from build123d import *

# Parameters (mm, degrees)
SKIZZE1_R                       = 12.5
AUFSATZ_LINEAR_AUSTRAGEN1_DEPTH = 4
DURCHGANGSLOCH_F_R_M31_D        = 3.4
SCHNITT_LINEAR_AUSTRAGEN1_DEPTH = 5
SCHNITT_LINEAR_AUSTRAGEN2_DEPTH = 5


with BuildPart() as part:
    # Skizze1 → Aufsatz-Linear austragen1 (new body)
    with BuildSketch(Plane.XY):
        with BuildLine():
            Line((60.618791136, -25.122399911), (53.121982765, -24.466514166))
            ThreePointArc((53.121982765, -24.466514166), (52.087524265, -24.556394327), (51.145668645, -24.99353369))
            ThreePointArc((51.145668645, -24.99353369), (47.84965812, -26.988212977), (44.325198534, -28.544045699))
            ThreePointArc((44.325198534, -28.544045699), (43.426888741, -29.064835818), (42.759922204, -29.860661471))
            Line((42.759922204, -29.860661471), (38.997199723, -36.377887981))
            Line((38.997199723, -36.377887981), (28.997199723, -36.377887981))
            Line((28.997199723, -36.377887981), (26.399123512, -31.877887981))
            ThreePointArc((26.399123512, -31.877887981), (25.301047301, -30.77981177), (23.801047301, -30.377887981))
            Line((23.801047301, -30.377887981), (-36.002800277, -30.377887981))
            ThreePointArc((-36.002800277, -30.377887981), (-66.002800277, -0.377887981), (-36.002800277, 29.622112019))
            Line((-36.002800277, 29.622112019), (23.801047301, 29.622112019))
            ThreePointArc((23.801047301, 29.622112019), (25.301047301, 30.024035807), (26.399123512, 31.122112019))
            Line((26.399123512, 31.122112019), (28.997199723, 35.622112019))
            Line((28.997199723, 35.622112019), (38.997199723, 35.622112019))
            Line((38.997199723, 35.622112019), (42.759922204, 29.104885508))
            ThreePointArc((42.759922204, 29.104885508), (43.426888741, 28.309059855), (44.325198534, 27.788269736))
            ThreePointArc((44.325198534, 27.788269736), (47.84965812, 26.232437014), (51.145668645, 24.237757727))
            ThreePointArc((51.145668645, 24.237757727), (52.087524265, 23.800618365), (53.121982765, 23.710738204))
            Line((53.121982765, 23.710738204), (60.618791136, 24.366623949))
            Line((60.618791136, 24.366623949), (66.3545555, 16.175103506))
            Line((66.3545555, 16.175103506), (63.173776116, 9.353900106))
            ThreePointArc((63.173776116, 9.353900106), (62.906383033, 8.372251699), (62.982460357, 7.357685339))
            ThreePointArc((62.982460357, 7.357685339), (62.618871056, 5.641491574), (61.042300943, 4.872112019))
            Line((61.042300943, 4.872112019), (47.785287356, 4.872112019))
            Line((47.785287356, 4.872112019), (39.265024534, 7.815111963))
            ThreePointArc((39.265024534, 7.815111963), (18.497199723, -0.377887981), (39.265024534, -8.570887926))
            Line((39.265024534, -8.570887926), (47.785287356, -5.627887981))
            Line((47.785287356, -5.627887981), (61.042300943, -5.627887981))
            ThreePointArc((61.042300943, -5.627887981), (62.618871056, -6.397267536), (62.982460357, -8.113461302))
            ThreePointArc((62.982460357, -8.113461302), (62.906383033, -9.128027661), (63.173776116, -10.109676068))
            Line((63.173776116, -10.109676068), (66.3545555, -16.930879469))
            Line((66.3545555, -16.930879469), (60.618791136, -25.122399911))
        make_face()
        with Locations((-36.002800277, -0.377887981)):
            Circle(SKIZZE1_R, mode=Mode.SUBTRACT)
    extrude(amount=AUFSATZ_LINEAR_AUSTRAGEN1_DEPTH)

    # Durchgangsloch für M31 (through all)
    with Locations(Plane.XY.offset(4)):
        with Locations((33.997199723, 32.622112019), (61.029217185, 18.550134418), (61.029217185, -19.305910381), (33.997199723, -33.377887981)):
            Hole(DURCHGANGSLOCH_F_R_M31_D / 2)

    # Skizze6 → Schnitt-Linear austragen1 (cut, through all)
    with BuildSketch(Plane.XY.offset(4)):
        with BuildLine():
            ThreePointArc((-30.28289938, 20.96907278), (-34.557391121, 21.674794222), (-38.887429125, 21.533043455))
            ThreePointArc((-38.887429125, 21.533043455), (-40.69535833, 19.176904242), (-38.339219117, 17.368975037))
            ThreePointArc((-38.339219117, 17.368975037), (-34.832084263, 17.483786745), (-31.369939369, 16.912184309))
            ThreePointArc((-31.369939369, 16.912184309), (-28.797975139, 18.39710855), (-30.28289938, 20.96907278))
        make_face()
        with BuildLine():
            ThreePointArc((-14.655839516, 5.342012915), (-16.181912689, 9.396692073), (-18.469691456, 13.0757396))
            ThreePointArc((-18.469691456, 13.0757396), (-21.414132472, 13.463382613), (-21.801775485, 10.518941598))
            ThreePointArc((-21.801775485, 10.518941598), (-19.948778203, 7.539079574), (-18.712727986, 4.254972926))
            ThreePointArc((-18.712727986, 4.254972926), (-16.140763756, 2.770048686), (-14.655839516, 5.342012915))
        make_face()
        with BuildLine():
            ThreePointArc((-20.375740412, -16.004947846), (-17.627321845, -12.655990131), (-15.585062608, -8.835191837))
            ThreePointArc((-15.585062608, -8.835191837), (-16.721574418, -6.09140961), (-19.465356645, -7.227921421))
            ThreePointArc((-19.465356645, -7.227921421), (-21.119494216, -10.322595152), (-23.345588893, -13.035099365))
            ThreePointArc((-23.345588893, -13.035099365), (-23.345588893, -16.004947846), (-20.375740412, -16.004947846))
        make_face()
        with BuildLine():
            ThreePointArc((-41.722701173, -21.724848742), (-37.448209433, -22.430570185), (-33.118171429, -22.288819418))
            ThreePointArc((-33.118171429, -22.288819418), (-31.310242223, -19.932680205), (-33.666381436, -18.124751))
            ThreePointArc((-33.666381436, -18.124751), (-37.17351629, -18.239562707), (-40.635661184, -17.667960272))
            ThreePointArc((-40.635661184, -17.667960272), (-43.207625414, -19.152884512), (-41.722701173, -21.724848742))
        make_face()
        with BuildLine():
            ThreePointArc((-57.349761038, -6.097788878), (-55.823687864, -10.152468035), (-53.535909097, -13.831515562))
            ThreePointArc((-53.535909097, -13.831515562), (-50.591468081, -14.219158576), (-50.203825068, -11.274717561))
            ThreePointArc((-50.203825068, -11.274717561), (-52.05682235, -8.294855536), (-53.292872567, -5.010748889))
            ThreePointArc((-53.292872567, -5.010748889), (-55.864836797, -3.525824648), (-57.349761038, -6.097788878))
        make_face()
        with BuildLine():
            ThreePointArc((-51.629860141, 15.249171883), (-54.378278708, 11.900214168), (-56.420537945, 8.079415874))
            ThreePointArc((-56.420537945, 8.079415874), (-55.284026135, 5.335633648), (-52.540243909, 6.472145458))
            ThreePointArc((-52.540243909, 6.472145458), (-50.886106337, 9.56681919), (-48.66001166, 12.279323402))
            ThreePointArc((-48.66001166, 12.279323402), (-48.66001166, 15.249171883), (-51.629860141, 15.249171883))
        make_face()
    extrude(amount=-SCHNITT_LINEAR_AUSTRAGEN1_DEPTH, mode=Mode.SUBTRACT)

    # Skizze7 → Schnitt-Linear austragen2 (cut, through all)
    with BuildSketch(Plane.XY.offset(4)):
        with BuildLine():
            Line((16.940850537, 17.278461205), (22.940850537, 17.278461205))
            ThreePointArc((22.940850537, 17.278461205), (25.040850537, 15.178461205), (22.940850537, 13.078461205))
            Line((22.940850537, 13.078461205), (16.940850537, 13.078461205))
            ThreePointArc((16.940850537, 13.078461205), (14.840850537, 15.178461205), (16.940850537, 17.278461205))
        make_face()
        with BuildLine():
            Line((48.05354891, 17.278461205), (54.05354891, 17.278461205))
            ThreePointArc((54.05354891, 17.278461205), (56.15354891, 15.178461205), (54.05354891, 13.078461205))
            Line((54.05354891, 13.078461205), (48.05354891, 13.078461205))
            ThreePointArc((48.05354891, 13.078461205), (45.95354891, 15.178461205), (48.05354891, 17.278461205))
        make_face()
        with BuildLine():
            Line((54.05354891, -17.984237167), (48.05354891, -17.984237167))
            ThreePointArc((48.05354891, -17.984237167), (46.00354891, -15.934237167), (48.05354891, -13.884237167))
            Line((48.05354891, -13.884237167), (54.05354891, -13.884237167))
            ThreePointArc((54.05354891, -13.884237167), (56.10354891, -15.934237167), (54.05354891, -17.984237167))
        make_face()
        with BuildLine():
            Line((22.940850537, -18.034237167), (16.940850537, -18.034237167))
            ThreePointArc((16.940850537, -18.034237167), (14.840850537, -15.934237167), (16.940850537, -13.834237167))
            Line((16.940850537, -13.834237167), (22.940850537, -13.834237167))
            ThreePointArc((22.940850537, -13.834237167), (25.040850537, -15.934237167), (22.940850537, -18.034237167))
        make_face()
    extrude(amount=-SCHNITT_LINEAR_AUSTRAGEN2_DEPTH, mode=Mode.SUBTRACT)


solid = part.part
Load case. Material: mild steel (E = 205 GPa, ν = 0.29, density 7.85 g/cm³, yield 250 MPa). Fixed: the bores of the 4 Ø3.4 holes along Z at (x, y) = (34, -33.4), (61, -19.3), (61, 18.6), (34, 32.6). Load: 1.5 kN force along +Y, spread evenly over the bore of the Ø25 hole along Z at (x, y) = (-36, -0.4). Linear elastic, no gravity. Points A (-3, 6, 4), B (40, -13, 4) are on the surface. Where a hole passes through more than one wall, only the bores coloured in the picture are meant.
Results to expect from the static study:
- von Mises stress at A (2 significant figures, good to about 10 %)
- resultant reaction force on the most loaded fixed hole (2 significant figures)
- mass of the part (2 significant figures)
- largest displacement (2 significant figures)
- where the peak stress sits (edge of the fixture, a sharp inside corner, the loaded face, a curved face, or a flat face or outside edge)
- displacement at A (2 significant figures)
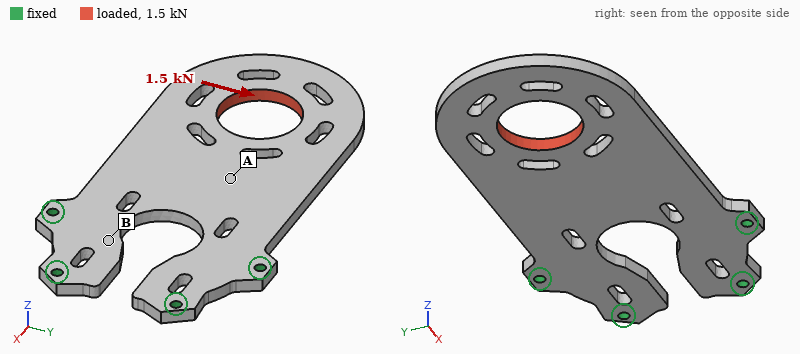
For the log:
20 MPa
1.6 kN
180 g
38 µm
a curved face
9.6 µm
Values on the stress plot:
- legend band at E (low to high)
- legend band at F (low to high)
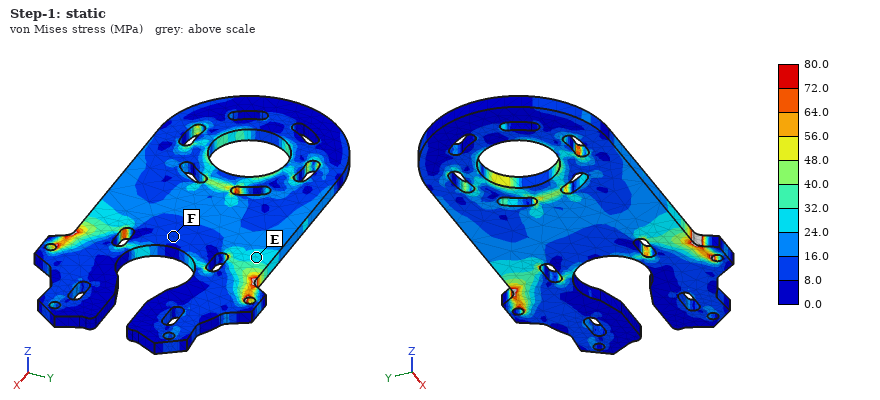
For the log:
24.0 to 32.0 MPa
8.0 to 16.0 MPa
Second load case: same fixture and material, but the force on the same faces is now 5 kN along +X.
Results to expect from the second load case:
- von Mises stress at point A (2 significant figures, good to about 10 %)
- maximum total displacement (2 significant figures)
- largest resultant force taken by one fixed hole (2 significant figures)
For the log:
13 MPa
20 µm
1.6 kN
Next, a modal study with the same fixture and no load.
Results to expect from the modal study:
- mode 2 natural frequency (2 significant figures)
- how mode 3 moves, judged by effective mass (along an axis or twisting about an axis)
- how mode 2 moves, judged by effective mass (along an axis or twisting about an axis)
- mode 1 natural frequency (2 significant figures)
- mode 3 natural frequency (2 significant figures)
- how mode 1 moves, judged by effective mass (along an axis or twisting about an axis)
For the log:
1300 Hz
along Z
twisting about X
330 Hz
1800 Hz
along Z
